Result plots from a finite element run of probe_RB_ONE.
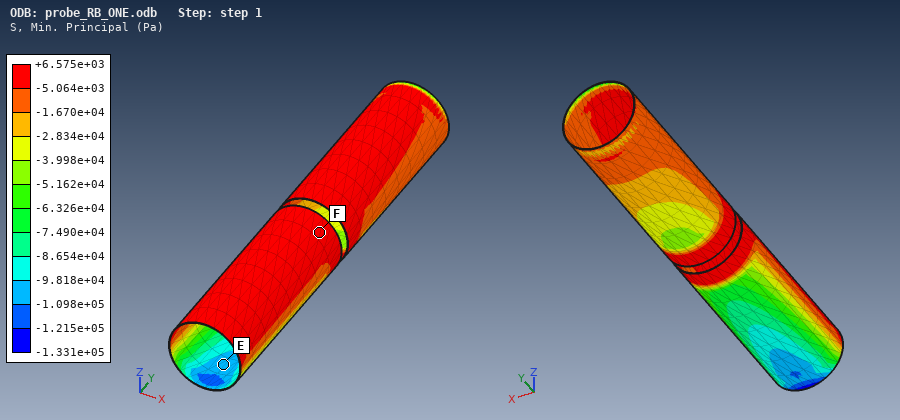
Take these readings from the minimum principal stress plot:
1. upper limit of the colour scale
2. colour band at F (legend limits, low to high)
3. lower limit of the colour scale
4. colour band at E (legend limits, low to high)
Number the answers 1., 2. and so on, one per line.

1. +6.575e+03 Pa
2. -5.064e+03 to +6.575e+03 Pa
3. -1.331e+05 Pa
4. -1.098e+05 to -9.818e+04 Pa
